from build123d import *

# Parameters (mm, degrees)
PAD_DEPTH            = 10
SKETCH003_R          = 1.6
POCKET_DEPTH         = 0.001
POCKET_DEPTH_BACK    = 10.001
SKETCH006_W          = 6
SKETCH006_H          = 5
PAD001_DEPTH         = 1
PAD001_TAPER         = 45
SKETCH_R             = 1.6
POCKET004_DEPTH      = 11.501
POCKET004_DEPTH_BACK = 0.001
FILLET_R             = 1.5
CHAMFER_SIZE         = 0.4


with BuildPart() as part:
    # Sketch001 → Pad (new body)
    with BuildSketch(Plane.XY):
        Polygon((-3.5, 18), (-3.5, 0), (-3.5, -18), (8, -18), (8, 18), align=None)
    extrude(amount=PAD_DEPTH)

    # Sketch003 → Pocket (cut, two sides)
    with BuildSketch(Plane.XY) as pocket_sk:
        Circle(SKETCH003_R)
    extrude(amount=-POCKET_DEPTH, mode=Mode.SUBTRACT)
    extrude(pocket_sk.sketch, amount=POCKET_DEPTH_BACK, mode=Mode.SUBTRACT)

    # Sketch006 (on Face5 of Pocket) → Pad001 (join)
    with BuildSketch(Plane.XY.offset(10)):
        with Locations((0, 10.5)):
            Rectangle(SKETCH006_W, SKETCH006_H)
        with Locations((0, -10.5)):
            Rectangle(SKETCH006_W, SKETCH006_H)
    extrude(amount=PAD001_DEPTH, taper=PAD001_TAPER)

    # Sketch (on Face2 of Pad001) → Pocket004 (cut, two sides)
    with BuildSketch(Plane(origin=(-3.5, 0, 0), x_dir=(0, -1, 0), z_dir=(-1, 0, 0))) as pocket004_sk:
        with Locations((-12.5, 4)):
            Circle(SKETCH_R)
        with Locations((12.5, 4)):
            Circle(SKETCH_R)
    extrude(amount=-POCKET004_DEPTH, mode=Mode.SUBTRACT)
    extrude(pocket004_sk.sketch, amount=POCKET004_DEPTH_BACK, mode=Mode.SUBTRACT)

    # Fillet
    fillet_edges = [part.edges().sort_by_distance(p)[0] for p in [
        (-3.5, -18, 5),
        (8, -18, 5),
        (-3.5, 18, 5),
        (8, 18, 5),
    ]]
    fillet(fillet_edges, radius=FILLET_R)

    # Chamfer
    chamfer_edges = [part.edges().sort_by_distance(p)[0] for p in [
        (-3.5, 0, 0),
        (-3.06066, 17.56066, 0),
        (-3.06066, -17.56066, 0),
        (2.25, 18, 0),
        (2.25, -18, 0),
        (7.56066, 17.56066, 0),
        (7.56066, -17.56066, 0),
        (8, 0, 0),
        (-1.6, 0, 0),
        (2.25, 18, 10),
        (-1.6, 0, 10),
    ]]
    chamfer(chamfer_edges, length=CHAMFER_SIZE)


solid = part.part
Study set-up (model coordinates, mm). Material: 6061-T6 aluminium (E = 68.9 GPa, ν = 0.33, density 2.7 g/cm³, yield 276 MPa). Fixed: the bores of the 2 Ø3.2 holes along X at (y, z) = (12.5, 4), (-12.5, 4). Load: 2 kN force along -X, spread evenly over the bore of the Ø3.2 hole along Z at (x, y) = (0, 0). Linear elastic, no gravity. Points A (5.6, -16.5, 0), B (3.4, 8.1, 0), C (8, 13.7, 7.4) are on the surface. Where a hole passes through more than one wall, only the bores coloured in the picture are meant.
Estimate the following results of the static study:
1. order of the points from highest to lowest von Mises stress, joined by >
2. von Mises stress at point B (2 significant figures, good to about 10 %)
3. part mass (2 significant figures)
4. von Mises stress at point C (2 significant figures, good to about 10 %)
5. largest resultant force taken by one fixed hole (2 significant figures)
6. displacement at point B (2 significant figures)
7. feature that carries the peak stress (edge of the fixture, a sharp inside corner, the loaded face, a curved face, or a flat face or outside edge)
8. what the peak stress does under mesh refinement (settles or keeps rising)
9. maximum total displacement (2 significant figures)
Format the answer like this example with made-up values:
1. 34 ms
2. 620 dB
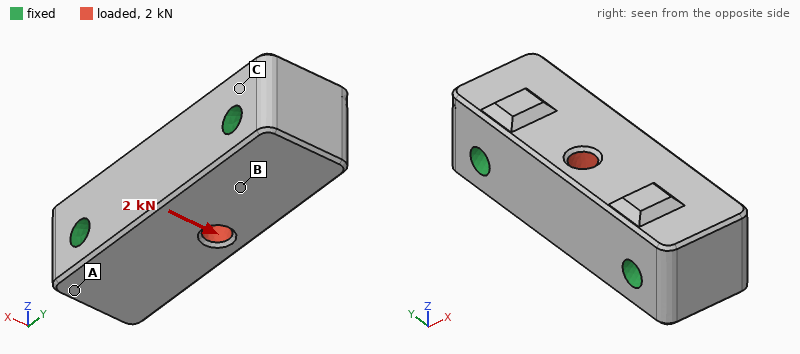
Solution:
1. B > C > A
2. 22 MPa
3. 10 g
4. 10 MPa
5. 1.0 kN
6. 1.9 µm
7. edge of the fixture
8. keeps rising
9. 7.6 µm
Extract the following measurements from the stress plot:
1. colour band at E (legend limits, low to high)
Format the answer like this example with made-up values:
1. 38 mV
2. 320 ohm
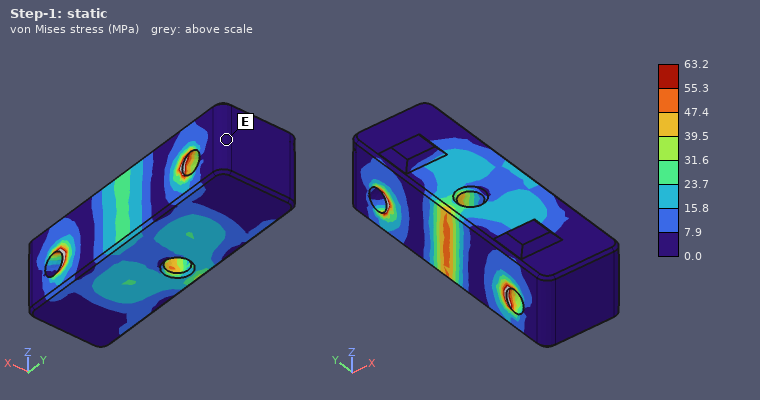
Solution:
1. 0.0 to 7.9 MPa
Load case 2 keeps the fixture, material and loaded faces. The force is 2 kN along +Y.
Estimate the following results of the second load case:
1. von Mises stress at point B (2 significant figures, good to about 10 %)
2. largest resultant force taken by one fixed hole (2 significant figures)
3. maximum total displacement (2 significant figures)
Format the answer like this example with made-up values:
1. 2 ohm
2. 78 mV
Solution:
1. 8.0 MPa
2. 1.0 kN
3. 2.7 µm
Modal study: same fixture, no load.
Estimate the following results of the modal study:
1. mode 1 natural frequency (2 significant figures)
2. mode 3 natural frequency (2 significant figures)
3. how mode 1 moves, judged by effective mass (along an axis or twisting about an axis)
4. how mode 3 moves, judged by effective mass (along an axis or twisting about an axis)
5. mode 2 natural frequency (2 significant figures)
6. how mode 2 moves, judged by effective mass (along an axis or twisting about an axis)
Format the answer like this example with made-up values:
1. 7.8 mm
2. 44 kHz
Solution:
1. 42 kHz
2. 60 kHz
3. along Z
4. twisting about Y
5. 51 kHz
6. along X
